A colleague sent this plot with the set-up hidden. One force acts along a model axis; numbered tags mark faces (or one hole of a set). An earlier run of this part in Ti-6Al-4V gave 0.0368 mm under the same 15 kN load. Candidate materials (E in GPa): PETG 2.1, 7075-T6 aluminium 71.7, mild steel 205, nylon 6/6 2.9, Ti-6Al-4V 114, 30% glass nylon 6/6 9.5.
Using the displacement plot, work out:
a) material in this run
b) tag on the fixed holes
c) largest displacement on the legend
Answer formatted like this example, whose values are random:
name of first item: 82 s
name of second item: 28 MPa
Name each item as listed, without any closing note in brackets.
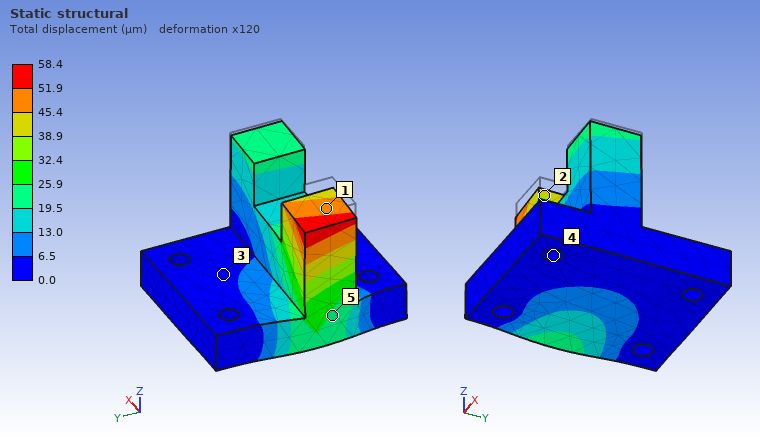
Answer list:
material in this run: 7075-T6 aluminium
tag on the fixed holes: 4
largest displacement on the legend: 58.4 µm
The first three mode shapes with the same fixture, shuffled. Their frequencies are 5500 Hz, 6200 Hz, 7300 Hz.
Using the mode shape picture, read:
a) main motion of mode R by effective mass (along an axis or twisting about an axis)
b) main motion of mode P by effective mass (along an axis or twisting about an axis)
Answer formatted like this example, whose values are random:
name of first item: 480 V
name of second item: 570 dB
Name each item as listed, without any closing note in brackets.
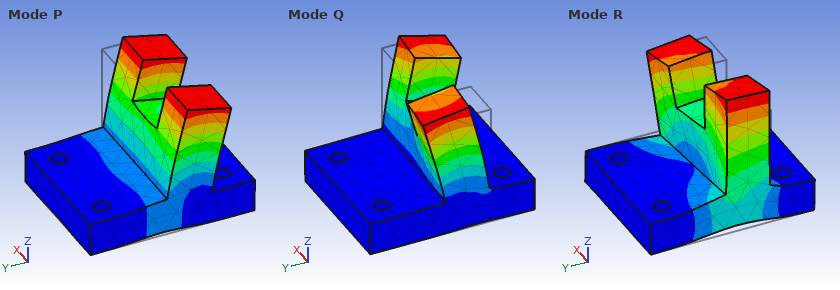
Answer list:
main motion of mode R by effective mass: along X
main motion of mode P by effective mass: along Y
